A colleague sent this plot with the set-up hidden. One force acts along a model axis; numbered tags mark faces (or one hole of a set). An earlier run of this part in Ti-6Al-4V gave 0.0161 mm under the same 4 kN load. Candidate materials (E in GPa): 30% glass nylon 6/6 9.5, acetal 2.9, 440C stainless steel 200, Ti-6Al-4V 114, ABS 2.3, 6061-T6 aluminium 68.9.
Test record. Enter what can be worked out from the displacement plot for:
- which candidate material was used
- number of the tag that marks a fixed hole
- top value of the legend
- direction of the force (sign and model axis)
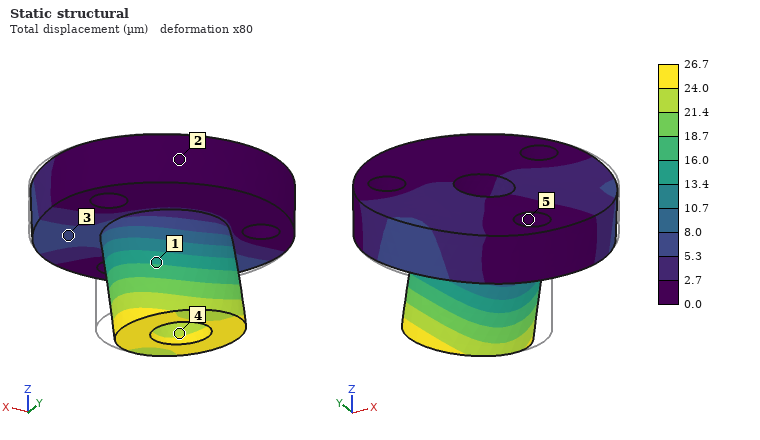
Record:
6061-T6 aluminium
5
26.7 µm
-X
